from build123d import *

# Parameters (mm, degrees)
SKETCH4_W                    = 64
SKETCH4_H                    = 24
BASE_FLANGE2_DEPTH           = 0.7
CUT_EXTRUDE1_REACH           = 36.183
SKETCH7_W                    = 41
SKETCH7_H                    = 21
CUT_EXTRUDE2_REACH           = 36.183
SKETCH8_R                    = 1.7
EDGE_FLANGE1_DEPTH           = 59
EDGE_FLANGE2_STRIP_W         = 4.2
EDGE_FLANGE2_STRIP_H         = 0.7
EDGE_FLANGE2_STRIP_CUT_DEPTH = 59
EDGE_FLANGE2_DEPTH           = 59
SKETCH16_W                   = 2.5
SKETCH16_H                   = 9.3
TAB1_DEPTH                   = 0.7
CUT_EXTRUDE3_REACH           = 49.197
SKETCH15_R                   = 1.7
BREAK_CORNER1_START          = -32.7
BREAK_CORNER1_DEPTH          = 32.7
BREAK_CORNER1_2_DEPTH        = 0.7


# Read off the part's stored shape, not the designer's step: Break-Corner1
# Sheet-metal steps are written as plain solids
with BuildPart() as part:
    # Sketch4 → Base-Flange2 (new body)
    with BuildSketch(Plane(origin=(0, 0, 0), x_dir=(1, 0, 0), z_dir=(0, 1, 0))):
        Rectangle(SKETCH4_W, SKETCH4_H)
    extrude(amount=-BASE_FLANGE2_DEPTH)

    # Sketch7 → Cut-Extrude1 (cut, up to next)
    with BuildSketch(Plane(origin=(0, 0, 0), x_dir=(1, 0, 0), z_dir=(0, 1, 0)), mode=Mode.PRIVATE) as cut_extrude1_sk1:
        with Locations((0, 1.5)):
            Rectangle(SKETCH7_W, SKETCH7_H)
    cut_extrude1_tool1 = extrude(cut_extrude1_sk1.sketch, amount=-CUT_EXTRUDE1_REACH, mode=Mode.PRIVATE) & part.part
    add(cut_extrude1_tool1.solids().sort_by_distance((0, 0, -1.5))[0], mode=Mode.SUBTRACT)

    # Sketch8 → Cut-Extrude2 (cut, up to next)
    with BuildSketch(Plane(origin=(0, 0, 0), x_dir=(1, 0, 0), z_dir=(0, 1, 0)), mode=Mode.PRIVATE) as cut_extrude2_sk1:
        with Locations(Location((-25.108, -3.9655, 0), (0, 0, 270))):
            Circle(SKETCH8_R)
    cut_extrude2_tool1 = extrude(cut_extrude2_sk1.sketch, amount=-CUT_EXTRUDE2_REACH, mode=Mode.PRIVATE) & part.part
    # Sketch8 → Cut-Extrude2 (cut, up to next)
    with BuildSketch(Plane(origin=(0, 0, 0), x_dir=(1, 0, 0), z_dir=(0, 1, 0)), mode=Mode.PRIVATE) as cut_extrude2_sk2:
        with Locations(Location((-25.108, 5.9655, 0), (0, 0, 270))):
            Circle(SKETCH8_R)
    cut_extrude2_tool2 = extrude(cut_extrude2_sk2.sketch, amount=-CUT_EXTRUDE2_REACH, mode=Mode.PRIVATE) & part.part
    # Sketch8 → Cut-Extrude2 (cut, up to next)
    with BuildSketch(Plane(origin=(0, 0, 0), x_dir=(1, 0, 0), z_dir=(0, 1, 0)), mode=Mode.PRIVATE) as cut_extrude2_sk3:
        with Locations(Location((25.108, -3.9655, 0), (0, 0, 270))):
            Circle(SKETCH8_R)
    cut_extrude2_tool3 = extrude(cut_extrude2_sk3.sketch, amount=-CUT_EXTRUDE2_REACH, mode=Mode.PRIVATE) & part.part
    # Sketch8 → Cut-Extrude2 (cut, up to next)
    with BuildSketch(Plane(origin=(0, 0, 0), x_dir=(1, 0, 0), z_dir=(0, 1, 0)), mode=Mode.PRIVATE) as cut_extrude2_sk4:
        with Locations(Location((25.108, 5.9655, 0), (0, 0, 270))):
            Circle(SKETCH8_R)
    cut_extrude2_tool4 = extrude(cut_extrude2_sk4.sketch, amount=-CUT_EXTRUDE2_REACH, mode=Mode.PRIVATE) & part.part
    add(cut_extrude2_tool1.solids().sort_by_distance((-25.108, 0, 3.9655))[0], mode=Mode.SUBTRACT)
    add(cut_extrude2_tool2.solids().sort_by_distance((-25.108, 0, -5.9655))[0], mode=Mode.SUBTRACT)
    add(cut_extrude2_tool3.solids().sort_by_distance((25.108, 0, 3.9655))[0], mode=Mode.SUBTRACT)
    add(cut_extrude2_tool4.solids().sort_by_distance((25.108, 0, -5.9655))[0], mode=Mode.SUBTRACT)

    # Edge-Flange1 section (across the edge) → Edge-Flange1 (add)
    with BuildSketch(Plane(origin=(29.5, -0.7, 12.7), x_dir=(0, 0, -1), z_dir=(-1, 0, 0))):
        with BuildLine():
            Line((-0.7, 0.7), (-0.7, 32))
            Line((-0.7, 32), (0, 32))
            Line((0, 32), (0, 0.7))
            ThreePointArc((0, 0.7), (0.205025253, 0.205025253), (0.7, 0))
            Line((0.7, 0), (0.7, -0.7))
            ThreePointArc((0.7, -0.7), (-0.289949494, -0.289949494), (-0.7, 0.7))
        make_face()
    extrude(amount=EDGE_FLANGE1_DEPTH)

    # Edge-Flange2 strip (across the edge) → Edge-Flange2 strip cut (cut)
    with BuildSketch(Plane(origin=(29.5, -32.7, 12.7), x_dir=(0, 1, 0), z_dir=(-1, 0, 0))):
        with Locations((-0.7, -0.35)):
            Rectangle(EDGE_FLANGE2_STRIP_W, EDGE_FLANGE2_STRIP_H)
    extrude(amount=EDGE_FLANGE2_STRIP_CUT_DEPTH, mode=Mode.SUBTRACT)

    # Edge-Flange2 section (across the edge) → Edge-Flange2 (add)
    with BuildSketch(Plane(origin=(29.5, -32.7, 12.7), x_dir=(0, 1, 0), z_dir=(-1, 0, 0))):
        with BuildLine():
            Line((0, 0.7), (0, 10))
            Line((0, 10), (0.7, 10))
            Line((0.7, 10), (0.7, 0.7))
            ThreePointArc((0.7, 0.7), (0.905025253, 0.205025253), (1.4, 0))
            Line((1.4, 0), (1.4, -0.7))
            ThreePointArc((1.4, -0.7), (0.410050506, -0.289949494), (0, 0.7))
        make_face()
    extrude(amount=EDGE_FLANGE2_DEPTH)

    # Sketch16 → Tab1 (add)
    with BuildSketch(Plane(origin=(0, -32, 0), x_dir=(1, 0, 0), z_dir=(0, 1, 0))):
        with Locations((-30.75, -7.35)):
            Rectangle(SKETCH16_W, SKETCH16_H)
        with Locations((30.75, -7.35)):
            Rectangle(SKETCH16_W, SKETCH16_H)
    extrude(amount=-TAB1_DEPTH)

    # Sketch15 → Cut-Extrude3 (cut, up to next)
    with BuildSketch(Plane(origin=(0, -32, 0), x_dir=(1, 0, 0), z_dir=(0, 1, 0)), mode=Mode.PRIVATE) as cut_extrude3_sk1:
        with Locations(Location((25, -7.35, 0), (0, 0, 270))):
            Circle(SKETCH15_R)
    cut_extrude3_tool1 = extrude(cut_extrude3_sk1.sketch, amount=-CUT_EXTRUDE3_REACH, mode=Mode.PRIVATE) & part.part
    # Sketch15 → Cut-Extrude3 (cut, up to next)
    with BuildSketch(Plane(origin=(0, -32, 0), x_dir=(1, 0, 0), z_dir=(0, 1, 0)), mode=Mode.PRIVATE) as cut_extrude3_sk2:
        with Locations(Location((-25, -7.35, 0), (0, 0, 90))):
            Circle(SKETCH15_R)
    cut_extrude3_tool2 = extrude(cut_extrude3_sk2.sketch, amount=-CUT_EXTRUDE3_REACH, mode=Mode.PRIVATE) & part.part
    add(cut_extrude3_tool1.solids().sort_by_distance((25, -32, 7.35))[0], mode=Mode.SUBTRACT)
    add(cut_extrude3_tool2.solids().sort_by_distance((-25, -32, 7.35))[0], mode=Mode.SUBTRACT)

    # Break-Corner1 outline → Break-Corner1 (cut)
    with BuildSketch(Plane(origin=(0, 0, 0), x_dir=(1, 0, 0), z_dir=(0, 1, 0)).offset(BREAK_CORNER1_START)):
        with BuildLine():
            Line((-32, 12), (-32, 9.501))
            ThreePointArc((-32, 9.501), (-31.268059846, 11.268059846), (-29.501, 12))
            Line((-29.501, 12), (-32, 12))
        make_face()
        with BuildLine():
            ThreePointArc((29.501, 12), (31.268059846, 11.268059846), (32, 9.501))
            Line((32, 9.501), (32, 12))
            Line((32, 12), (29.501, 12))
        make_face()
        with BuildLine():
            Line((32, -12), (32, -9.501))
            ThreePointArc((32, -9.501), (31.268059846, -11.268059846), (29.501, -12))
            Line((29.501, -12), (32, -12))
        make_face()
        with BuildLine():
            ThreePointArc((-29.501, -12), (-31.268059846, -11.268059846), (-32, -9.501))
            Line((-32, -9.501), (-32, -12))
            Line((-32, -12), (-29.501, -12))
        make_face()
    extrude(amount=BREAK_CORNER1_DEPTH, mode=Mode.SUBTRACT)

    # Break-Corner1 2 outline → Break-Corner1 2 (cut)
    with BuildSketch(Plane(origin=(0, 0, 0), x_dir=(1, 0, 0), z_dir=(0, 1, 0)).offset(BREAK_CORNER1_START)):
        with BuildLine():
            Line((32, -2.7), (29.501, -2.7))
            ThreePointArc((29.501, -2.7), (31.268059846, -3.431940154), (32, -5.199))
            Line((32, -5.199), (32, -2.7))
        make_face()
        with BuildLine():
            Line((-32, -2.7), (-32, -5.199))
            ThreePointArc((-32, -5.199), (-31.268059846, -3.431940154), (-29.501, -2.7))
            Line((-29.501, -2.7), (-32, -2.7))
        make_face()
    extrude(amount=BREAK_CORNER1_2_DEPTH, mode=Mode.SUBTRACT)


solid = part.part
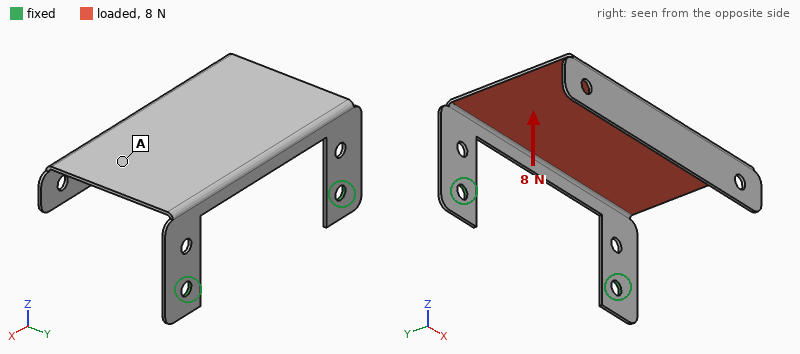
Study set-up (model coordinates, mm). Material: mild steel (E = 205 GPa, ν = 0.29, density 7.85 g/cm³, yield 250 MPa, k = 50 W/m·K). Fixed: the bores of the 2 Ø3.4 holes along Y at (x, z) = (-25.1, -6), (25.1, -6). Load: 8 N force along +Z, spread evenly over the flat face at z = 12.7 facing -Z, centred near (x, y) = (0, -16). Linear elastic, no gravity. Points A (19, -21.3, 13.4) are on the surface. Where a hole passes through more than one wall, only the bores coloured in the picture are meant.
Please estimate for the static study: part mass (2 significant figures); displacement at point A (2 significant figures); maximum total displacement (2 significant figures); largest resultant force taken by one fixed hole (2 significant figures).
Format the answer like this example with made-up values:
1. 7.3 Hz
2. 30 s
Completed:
1. 17 g
2. 0.49 mm
3. 0.74 mm
4. 4.2 N
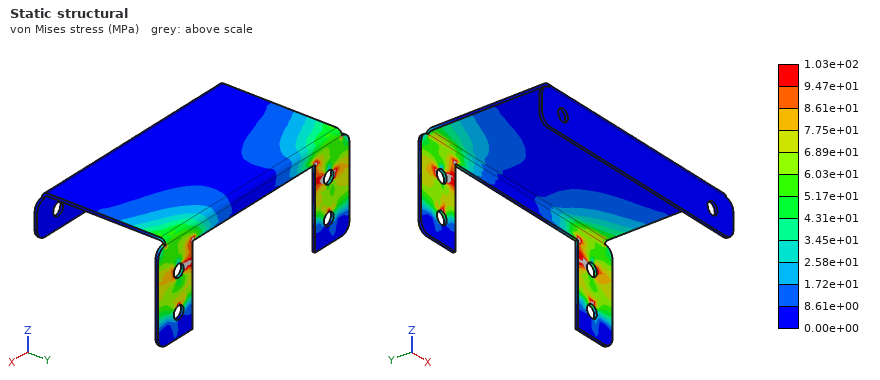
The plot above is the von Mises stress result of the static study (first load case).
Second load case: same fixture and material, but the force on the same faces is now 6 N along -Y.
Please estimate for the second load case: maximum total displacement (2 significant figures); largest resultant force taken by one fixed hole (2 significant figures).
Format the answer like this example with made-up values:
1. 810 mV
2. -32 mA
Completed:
1. 0.25 mm
2. 3.0 N
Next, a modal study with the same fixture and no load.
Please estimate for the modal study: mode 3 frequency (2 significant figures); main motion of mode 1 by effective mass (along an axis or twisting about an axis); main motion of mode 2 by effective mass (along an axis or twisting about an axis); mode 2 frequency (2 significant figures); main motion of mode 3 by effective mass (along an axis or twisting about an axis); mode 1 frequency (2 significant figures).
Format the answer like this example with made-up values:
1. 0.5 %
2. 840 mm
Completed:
1. 540 Hz
2. along Z
3. along X
4. 400 Hz
5. along Y
6. 140 Hz
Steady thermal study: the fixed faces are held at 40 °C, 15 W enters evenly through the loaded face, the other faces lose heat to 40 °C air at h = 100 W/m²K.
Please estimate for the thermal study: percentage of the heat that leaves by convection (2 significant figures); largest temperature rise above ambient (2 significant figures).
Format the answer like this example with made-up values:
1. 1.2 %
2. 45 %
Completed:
1. 95 %
2. 49 K
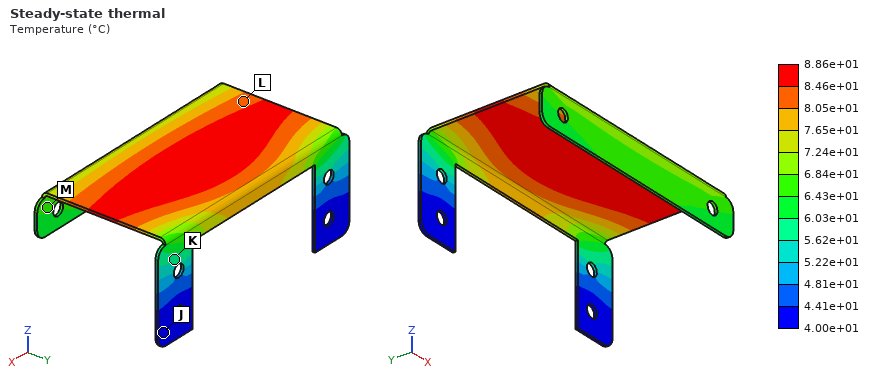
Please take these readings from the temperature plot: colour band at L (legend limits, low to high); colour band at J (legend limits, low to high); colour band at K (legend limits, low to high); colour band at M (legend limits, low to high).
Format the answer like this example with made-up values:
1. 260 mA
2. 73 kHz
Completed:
1. 8.05e+01 to 8.46e+01 °C
2. 4.00e+01 to 4.41e+01 °C
3. 5.62e+01 to 6.03e+01 °C
4. 6.43e+01 to 6.84e+01 °C
